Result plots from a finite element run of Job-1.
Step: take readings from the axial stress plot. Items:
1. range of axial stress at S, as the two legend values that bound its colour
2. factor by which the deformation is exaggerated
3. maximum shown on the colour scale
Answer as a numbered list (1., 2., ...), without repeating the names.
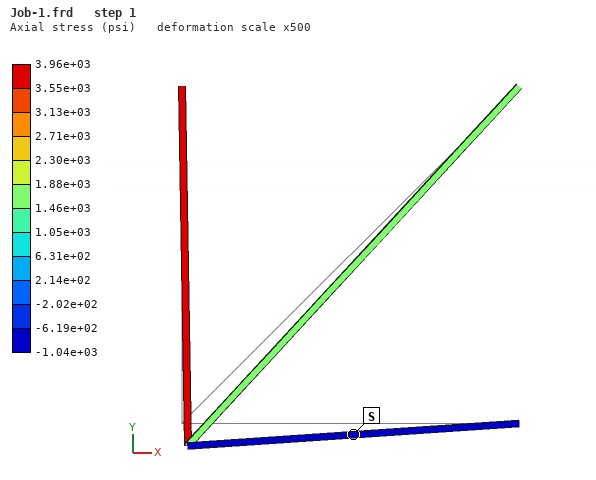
1. -1.04e+03 to -6.19e+02 psi
2. 500
3. 3.96e+03 psi
